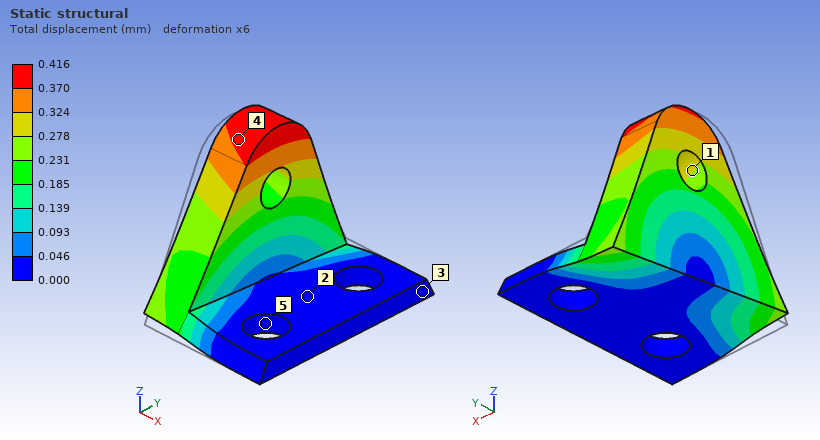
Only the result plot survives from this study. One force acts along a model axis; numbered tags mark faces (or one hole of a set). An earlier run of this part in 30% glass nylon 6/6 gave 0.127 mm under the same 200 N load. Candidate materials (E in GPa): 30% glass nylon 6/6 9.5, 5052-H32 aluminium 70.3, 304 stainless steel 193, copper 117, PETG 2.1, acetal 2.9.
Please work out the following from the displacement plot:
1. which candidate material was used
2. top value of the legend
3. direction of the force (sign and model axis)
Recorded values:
acetal
0.416 mm
+Y
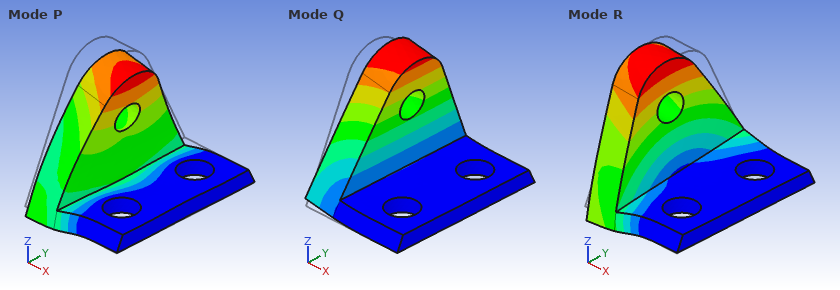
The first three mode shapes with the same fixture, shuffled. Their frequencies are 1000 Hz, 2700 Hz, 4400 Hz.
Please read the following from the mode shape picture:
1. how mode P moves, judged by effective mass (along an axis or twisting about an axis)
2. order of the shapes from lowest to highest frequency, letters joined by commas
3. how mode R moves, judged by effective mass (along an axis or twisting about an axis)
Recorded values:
along Z
Q, R, P
along Y
